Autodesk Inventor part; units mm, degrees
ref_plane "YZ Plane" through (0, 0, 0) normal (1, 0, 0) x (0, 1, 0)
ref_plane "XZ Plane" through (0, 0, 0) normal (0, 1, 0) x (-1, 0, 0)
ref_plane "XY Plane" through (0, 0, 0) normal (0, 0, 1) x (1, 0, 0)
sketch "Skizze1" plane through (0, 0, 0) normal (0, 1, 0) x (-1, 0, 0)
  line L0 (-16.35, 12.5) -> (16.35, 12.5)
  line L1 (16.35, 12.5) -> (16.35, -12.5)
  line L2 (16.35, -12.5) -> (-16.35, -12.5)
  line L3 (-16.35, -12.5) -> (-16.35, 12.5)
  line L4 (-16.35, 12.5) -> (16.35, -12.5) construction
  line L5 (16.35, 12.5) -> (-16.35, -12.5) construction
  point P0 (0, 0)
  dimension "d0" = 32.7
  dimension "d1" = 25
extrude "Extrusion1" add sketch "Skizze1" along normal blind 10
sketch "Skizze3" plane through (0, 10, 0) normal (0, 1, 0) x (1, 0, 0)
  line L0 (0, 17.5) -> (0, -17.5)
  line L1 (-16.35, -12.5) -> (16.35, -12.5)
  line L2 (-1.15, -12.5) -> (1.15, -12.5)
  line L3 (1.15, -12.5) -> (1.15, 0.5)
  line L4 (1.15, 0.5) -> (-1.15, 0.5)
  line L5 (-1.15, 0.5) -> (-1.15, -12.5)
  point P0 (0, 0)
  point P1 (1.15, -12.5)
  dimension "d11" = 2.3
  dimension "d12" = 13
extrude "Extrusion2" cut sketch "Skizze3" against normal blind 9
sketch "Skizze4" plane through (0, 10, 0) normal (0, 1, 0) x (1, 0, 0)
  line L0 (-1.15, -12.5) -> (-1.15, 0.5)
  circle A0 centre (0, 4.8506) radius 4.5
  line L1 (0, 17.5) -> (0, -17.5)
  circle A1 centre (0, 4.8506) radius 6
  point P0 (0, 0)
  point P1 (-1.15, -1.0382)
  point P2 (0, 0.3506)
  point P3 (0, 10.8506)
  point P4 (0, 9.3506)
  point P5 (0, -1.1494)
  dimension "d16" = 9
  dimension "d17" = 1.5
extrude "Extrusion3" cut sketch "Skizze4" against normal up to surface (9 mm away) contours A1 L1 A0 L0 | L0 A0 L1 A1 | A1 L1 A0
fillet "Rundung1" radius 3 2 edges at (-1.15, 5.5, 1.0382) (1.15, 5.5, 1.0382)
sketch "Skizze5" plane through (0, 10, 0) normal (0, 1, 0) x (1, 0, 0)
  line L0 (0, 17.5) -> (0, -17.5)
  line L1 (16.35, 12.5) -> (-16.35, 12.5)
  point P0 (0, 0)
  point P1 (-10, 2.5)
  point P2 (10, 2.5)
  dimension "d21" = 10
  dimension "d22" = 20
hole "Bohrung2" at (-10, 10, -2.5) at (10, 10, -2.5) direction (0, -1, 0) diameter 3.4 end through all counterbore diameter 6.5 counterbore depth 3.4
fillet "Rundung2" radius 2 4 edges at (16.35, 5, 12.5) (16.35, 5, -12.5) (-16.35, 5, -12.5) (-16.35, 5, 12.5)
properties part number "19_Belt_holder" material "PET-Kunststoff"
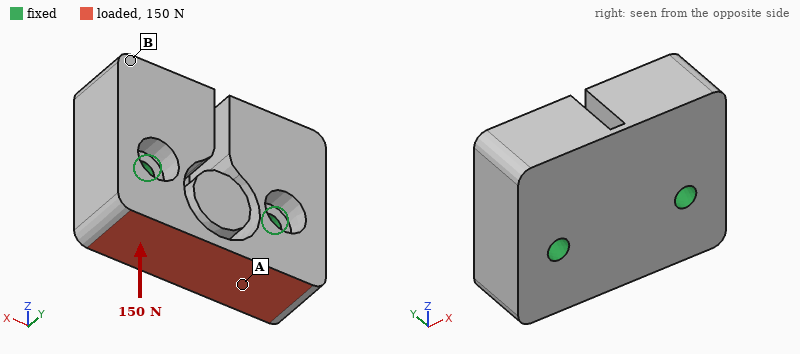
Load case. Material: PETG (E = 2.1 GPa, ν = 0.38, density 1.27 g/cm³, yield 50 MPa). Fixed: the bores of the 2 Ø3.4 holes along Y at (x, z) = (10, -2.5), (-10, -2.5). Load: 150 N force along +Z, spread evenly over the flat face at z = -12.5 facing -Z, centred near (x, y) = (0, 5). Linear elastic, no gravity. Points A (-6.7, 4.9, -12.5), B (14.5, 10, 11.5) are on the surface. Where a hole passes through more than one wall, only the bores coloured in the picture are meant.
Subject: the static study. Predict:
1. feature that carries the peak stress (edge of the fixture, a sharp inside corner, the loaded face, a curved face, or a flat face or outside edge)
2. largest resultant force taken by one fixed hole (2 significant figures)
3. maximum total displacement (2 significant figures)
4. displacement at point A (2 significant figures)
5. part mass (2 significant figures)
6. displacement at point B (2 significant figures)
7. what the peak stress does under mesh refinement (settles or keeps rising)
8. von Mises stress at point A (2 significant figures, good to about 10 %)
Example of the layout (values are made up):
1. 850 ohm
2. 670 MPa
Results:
1. edge of the fixture
2. 77 N
3. 27 µm
4. 10 µm
5. 9.0 g
6. 5.8 µm
7. keeps rising
8. 1.1 MPa
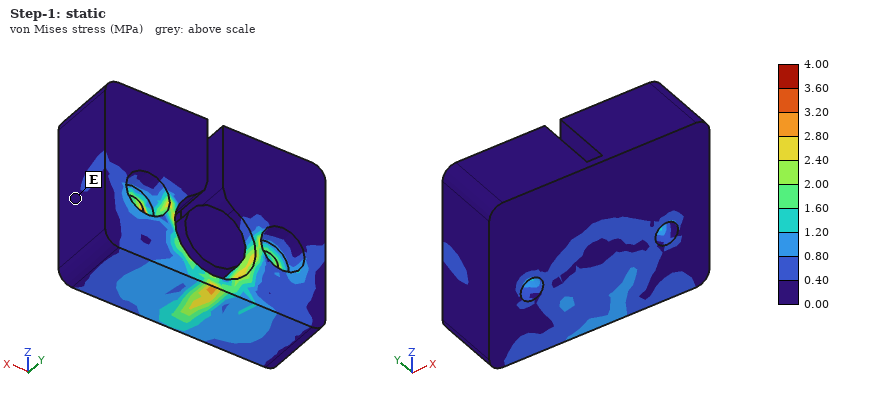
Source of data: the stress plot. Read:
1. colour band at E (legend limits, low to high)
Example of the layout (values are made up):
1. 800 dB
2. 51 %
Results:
1. 0.00 to 0.40 MPa
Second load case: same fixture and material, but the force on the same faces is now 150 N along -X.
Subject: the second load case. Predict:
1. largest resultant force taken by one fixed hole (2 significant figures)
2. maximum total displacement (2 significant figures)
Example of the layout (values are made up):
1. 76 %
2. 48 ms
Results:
1. 91 N
2. 28 µm
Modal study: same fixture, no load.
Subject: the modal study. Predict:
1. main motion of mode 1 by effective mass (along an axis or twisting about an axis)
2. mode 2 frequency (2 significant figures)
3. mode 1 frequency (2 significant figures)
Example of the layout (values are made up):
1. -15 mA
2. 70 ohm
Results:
1. along Y
2. 4900 Hz
3. 4300 Hz
